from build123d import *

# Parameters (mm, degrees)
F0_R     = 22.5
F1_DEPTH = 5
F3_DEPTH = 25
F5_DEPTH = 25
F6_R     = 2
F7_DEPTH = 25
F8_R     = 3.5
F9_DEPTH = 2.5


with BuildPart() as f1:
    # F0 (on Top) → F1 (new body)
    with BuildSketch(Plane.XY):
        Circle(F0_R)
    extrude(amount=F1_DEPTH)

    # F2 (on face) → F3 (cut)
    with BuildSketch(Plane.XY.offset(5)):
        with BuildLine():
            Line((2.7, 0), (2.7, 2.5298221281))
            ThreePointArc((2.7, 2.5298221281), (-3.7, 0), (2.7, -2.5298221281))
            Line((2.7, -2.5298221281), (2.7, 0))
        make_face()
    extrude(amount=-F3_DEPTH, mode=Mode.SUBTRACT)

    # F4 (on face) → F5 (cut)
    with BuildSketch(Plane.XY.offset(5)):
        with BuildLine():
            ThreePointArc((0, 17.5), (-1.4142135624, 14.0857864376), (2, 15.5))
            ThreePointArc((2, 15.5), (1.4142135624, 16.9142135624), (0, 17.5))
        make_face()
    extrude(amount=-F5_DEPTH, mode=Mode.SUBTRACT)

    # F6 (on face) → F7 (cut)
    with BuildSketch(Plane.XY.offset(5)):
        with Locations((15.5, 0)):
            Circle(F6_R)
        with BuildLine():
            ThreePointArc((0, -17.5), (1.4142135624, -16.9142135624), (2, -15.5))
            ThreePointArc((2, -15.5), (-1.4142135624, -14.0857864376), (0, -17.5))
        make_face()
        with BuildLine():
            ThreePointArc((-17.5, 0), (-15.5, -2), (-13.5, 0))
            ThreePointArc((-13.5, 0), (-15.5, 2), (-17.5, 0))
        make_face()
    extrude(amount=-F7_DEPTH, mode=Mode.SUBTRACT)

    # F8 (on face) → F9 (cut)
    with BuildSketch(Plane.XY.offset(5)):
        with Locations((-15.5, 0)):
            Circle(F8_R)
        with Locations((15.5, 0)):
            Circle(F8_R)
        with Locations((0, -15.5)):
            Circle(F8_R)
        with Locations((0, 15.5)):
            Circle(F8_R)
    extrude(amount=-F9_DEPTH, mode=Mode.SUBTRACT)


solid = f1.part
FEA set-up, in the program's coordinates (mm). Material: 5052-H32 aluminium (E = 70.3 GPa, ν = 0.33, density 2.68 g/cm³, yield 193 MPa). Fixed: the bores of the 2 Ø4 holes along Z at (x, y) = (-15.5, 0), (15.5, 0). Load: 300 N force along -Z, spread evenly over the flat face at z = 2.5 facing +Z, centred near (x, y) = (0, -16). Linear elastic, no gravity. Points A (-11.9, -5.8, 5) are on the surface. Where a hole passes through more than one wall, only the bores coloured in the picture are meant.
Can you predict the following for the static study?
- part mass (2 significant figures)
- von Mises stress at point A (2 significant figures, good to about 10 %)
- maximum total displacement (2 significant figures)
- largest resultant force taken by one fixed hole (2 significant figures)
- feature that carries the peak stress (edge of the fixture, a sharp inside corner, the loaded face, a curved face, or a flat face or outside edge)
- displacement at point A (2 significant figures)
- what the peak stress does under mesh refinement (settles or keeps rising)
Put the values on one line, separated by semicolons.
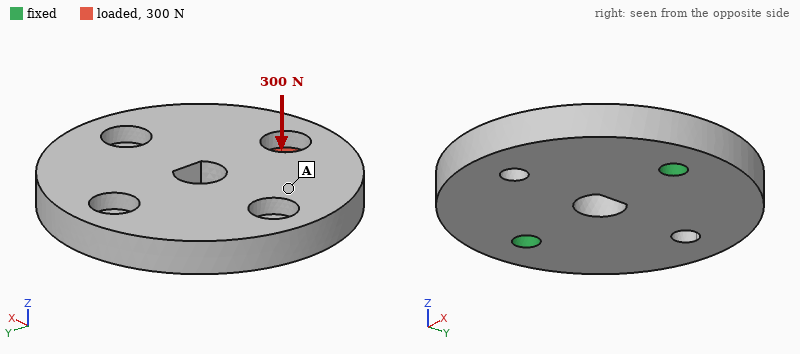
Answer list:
19 g; 16 MPa; 67 µm; 200 N; edge of the fixture; 14 µm; keeps rising
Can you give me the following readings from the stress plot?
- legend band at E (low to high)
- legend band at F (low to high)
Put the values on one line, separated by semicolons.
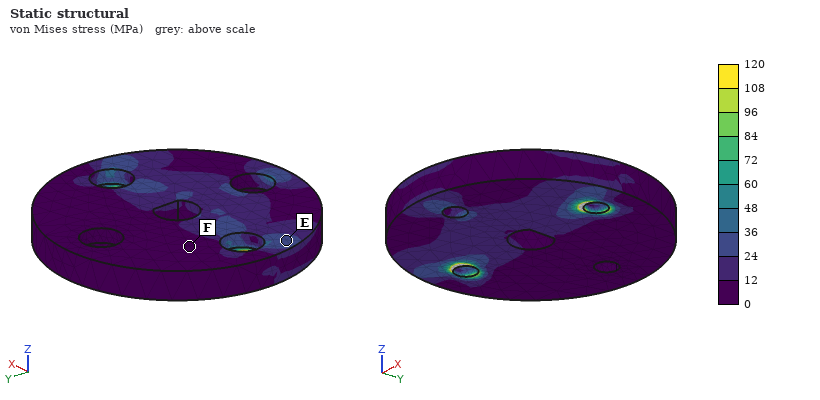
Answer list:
24 to 36 MPa; 0 to 12 MPa
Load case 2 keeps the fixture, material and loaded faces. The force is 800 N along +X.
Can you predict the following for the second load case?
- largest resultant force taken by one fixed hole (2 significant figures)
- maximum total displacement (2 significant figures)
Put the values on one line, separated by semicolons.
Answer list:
550 N; 6.6 µm
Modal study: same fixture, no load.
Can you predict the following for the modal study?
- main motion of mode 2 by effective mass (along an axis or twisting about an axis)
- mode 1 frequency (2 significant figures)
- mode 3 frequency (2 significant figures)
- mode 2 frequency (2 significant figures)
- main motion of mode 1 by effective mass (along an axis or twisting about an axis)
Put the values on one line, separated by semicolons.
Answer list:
along Z; 5100 Hz; 15 kHz; 8500 Hz; twisting about X
